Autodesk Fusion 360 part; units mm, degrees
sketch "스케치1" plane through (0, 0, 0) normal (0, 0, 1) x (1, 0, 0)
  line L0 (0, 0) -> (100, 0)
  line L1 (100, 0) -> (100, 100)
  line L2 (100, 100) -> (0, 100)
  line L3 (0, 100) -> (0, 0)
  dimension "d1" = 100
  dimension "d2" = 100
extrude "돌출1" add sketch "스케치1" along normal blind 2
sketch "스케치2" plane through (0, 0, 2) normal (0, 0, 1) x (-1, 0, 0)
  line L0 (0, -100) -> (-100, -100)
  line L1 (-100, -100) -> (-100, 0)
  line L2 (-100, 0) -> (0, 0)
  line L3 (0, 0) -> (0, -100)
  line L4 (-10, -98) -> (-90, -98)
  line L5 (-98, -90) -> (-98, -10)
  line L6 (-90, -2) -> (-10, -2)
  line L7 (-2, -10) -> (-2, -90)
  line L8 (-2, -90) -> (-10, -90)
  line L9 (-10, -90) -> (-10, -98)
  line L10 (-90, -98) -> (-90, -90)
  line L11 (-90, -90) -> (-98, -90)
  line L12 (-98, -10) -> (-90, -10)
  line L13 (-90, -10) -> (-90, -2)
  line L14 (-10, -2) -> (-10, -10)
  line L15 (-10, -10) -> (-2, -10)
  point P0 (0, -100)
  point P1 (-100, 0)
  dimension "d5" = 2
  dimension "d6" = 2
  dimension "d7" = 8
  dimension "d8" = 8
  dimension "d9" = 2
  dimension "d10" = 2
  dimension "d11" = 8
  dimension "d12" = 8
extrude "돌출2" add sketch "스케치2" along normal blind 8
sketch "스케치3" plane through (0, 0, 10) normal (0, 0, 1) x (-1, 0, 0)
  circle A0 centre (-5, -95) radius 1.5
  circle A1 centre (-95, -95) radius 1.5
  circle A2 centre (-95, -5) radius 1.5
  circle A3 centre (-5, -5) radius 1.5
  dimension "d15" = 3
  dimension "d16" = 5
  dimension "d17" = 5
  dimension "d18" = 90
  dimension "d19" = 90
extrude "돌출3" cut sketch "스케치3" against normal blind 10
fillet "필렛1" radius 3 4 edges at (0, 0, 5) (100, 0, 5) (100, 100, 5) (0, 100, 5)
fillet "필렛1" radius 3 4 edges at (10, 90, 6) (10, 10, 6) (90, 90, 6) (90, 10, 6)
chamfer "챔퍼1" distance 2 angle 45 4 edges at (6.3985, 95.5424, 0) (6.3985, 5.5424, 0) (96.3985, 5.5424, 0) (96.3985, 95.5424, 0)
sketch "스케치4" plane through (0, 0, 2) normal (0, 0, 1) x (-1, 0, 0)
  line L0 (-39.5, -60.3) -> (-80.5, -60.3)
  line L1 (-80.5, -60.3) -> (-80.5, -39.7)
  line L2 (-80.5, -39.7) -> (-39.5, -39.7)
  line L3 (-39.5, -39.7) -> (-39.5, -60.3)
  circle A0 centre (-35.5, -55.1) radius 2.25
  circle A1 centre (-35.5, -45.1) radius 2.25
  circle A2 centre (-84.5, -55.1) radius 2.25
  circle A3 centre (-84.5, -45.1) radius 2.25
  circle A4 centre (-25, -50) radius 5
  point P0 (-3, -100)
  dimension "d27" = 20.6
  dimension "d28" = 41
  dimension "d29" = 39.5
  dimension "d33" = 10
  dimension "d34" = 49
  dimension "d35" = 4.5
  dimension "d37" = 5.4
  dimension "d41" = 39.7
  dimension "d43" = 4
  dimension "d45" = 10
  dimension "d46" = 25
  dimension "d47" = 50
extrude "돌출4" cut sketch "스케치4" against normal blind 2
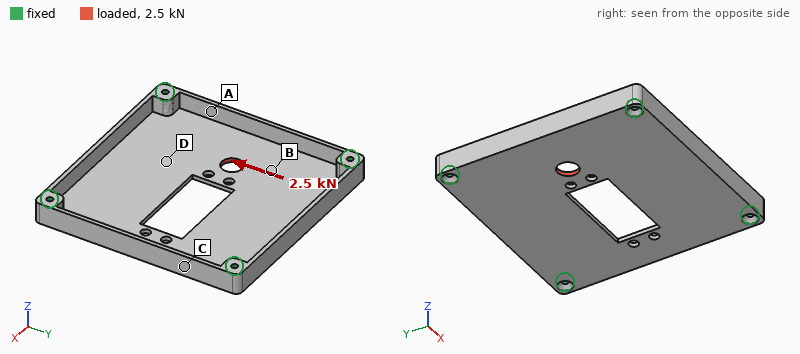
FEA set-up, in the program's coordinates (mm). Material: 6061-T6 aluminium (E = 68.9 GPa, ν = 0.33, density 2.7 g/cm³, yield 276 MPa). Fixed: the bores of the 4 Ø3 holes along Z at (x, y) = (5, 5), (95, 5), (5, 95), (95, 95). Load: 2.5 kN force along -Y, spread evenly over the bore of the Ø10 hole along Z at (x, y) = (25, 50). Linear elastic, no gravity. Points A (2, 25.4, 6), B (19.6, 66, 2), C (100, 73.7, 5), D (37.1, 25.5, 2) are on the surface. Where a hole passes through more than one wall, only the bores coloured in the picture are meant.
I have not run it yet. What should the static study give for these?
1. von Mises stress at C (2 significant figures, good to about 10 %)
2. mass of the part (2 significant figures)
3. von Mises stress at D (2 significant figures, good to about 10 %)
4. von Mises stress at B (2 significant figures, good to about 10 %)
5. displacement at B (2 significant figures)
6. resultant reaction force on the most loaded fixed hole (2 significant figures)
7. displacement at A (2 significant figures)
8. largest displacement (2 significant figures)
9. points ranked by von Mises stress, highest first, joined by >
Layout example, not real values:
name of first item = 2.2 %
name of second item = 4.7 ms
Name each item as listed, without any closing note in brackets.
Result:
von Mises stress at C = 4.0 MPa
mass of the part = 70 g
von Mises stress at D = 8.5 MPa
von Mises stress at B = 25 MPa
displacement at B = 14 µm
resultant reaction force on the most loaded fixed hole = 1.1 kN
displacement at A = 5.4 µm
largest displacement = 21 µm
points ranked by von Mises stress, highest first, joined by > = B > A > D > C
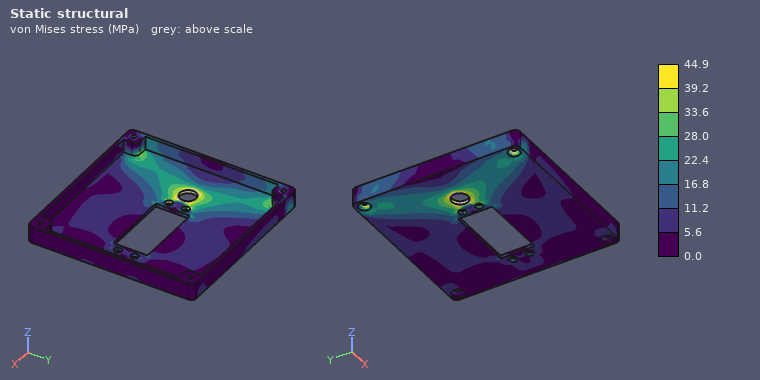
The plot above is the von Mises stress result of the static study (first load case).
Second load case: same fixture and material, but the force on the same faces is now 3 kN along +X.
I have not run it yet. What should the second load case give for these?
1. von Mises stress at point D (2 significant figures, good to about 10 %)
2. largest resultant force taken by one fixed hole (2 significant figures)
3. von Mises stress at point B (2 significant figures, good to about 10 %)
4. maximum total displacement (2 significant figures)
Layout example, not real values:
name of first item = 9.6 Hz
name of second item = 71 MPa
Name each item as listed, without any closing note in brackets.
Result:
von Mises stress at point D = 16 MPa
largest resultant force taken by one fixed hole = 860 N
von Mises stress at point B = 32 MPa
maximum total displacement = 45 µm
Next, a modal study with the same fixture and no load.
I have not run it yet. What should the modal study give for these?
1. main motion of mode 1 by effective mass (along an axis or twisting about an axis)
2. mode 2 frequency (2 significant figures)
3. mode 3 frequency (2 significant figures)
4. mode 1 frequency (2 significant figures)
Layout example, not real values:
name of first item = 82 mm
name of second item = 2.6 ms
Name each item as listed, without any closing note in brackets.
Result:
main motion of mode 1 by effective mass = along Z
mode 2 frequency = 2200 Hz
mode 3 frequency = 2700 Hz
mode 1 frequency = 1200 Hz
